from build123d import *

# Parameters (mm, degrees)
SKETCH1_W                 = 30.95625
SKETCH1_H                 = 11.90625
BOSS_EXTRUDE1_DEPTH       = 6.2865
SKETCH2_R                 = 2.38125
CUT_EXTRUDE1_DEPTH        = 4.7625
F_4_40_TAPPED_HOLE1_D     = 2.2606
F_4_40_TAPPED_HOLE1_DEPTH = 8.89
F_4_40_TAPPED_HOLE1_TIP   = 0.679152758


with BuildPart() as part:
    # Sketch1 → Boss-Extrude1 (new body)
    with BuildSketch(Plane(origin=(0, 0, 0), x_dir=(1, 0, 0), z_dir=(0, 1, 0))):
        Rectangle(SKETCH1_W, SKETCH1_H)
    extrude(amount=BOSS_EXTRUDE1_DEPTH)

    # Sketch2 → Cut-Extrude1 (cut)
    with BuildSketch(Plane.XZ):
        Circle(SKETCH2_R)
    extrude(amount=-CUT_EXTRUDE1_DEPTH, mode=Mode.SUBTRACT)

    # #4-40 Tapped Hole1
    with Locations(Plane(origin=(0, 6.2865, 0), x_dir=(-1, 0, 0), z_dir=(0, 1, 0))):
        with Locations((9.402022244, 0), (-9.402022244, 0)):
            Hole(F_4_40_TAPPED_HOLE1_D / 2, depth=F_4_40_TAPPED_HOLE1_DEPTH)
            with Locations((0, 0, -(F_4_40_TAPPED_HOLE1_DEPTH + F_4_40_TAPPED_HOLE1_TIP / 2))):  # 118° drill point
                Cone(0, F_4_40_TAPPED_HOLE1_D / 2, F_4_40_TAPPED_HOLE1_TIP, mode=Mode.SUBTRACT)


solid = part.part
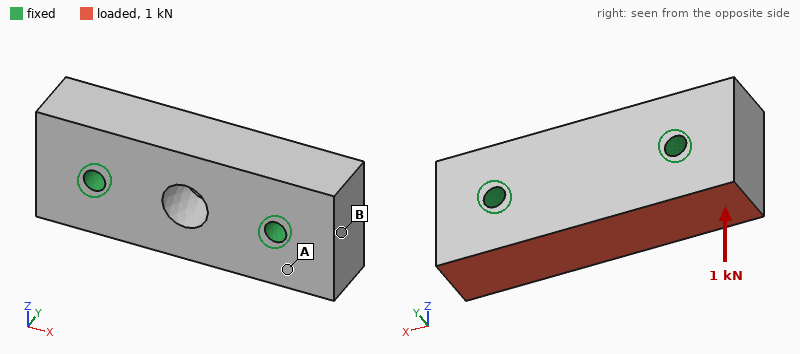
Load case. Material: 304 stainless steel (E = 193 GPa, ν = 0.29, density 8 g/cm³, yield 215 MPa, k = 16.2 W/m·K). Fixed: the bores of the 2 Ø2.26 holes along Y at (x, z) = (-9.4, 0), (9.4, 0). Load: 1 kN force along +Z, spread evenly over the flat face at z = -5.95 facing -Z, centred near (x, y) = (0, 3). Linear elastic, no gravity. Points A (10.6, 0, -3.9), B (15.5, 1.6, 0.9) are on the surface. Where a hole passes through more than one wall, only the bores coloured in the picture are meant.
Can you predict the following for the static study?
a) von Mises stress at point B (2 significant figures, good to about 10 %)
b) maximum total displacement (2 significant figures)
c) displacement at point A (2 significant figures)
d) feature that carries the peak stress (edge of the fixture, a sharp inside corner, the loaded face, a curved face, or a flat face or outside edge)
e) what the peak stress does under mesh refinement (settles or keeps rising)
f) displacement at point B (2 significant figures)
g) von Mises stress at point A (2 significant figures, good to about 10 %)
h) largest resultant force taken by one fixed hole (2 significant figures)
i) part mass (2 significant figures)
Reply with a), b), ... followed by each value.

a) 2.7 MPa
b) 0.58 µm
c) 0.15 µm
d) edge of the fixture
e) keeps rising
f) 0.14 µm
g) 6.8 MPa
h) 500 N
i) 17 g
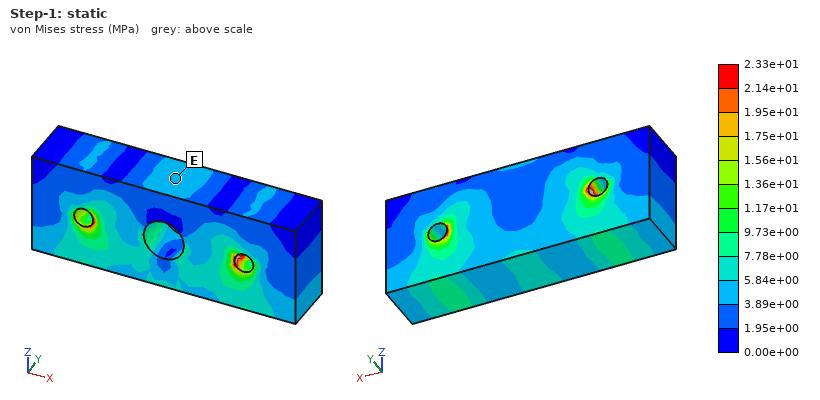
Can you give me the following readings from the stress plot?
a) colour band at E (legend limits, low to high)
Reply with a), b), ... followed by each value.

a) 3.89e+00 to 5.84e+00 MPa
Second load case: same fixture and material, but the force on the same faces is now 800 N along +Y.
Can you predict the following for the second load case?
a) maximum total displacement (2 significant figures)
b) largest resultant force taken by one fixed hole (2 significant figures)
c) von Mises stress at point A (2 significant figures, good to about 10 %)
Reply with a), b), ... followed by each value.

a) 2.3 µm
b) 400 N
c) 10 MPa
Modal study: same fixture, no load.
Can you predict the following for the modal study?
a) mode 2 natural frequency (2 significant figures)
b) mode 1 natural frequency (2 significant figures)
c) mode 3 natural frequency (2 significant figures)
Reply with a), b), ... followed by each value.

a) 52 kHz
b) 51 kHz
c) 54 kHz
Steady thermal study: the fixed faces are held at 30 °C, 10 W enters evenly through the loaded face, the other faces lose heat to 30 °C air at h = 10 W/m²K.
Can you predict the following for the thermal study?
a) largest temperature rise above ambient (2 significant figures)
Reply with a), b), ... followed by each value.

a) 32 K
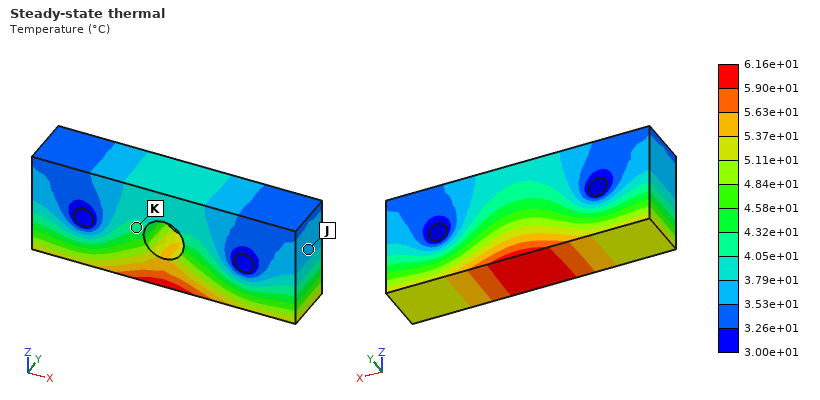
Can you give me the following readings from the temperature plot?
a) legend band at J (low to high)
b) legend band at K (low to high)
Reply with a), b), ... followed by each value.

a) 3.53e+01 to 3.79e+01 °C
b) 4.05e+01 to 4.32e+01 °C
